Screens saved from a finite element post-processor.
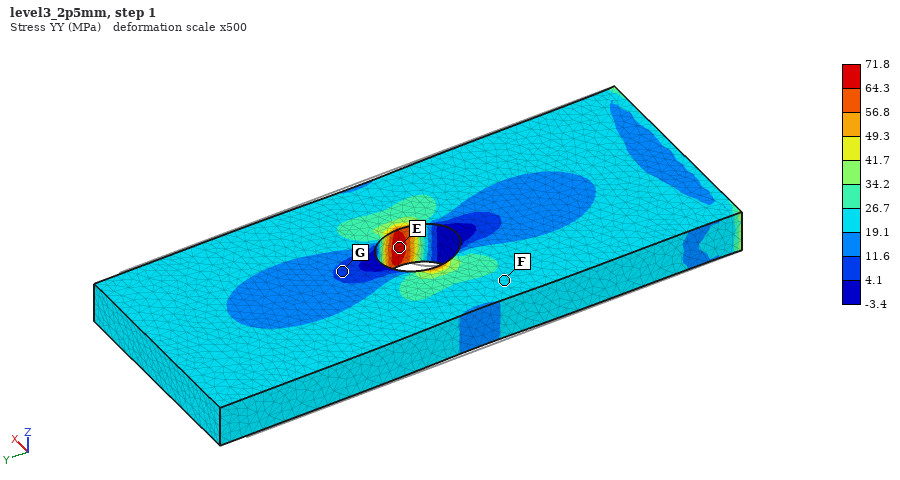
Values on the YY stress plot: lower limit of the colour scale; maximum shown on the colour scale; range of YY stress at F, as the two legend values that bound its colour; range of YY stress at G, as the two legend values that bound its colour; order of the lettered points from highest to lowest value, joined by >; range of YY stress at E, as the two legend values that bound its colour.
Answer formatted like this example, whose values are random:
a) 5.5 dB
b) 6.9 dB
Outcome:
a) -3.4 MPa
b) 71.8 MPa
c) 19.1 to 26.7 MPa
d) 4.1 to 11.6 MPa
e) E > F > G
f) 64.3 to 71.8 MPa
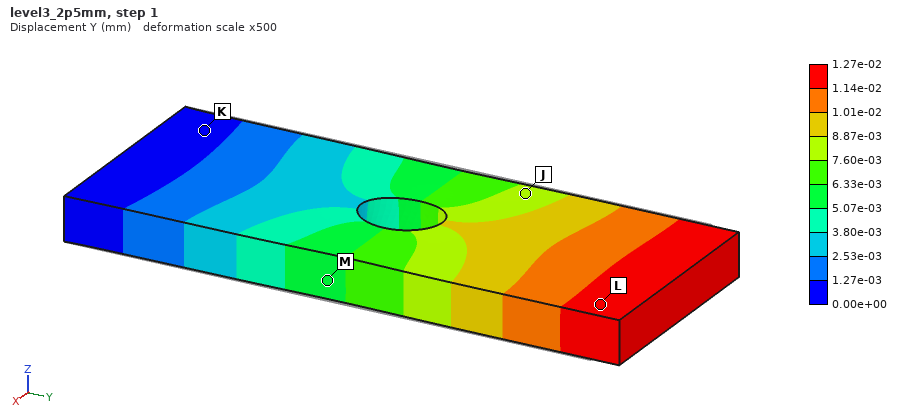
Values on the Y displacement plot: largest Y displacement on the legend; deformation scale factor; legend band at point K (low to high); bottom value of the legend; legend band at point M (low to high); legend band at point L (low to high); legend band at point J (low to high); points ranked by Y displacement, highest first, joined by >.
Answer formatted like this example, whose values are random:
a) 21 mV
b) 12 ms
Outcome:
a) 1.27e-02 mm
b) 500
c) 0.00e+00 to 1.27e-03 mm
d) 0.00e+00 mm
e) 5.07e-03 to 6.33e-03 mm
f) 1.14e-02 to 1.27e-02 mm
g) 7.60e-03 to 8.87e-03 mm
h) L > J > M > K
